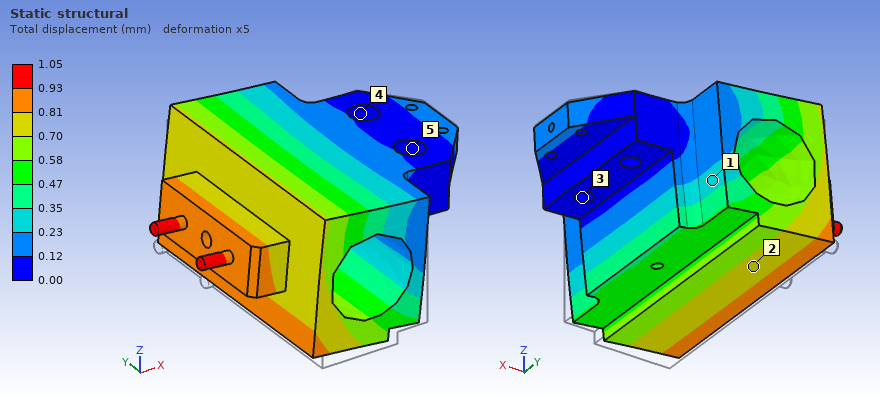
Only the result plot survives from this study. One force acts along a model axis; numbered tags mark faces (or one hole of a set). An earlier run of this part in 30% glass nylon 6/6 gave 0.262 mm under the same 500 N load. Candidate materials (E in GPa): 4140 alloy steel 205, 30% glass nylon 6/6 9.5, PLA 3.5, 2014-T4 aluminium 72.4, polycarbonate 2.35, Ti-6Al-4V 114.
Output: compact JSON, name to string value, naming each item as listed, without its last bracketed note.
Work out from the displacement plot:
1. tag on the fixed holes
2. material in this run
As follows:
{"tag on the fixed holes": "3", "material in this run": "polycarbonate"}
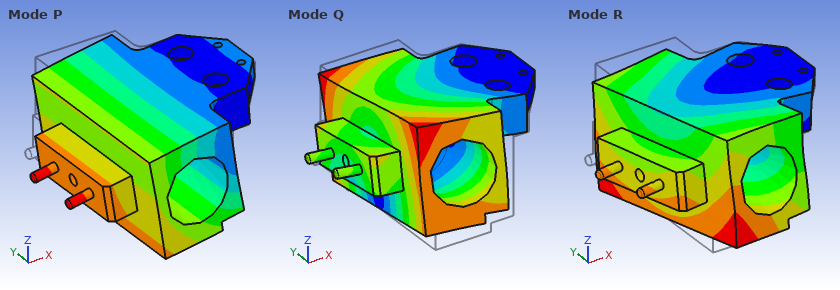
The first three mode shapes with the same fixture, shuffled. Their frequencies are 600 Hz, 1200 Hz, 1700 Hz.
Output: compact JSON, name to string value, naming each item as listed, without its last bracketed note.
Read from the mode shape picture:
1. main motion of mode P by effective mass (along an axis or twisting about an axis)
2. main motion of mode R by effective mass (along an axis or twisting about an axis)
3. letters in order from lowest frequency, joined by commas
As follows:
{"main motion of mode P by effective mass": "along Z", "main motion of mode R by effective mass": "along Y", "letters in order from lowest frequency, joined by commas": "P, R, Q"}
